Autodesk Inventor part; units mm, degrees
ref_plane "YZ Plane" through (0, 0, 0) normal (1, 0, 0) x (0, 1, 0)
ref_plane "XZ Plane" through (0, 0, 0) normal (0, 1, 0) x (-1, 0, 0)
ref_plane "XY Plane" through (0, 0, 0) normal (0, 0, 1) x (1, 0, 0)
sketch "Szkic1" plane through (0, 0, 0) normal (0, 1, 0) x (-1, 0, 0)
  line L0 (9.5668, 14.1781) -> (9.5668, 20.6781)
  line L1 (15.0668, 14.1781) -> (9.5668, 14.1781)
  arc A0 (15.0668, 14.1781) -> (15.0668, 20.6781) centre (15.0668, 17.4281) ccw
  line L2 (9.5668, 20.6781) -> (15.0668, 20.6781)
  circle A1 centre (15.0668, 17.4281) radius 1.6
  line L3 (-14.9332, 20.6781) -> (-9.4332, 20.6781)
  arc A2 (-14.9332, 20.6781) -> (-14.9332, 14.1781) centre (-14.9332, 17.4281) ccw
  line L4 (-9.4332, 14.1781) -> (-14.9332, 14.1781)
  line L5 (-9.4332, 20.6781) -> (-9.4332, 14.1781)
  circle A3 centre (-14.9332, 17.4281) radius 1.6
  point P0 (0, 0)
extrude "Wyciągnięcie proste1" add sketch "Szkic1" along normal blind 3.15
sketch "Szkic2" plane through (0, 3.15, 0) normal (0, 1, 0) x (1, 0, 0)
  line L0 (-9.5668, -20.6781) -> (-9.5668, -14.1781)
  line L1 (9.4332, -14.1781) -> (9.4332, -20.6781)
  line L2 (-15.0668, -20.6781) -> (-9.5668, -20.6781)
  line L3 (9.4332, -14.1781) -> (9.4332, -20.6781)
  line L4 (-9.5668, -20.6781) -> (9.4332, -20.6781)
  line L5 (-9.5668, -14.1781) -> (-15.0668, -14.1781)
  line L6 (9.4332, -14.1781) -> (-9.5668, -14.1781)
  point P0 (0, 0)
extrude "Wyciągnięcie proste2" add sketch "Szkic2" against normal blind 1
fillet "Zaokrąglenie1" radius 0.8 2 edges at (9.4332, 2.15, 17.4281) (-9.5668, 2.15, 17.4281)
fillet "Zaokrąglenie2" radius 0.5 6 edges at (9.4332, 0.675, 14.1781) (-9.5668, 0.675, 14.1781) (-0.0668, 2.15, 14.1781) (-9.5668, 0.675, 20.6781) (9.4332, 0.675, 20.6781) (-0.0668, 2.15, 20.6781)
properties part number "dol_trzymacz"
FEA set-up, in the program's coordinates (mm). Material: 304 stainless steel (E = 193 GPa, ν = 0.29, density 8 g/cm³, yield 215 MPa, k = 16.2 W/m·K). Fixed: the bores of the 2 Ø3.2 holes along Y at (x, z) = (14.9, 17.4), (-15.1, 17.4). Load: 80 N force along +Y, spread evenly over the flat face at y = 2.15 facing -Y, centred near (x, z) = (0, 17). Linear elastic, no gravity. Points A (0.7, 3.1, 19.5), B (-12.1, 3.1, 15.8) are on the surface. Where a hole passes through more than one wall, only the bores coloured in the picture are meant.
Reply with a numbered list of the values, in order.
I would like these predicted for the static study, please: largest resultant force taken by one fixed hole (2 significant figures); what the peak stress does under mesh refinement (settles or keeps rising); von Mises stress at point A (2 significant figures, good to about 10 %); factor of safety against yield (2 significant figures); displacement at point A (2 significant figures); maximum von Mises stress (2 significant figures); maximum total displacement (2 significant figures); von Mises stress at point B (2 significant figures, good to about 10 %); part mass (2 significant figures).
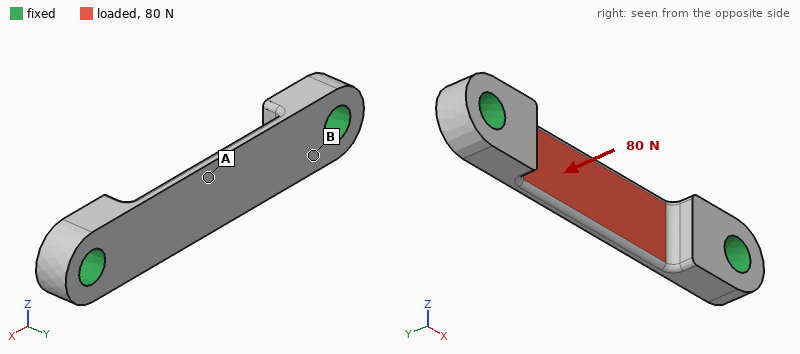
1. 56 N
2. settles
3. 71 MPa
4. 1.8
5. 18 µm
6. 120 MPa
7. 18 µm
8. 16 MPa
9. 3.2 g
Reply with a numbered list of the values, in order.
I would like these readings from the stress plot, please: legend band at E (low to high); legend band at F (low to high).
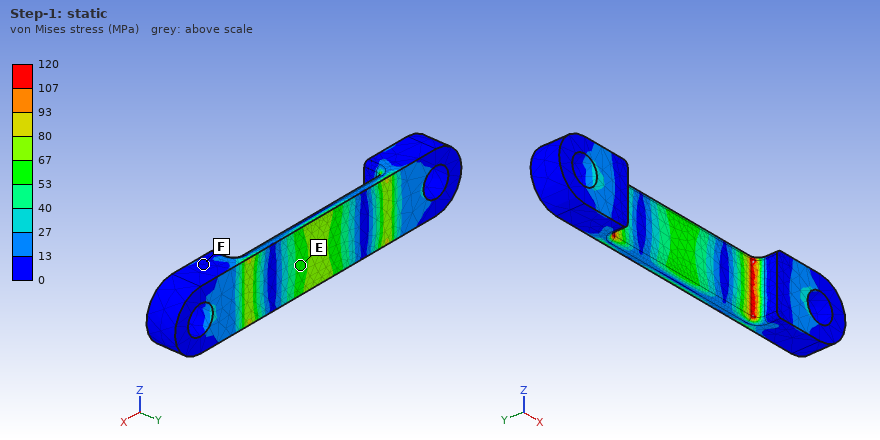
1. 53 to 67 MPa
2. 0 to 13 MPa
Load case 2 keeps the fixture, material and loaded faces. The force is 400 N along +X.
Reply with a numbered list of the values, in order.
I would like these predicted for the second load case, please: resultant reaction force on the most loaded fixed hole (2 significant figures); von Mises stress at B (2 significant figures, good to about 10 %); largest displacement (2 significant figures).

1. 200 N
2. 30 MPa
3. 1.9 µm
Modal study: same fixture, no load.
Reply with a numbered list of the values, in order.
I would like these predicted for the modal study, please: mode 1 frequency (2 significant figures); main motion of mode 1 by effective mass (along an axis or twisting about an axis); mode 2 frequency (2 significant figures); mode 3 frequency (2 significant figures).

1. 13 kHz
2. along Y
3. 27 kHz
4. 32 kHz
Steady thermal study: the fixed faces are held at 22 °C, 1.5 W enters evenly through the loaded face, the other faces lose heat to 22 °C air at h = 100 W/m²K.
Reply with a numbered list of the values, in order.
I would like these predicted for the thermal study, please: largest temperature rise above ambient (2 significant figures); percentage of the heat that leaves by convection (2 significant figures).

1. 35 K
2. 35 %
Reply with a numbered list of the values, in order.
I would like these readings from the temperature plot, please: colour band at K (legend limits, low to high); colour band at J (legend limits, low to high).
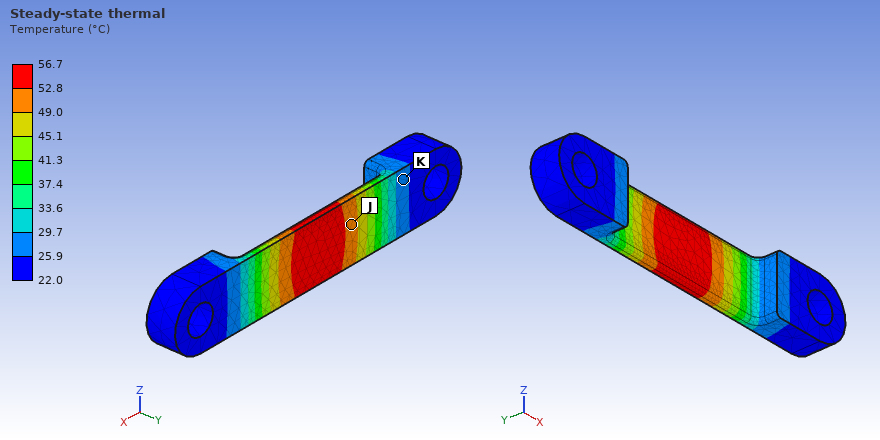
1. 25.9 to 29.7 °C
2. 49.0 to 52.8 °C
